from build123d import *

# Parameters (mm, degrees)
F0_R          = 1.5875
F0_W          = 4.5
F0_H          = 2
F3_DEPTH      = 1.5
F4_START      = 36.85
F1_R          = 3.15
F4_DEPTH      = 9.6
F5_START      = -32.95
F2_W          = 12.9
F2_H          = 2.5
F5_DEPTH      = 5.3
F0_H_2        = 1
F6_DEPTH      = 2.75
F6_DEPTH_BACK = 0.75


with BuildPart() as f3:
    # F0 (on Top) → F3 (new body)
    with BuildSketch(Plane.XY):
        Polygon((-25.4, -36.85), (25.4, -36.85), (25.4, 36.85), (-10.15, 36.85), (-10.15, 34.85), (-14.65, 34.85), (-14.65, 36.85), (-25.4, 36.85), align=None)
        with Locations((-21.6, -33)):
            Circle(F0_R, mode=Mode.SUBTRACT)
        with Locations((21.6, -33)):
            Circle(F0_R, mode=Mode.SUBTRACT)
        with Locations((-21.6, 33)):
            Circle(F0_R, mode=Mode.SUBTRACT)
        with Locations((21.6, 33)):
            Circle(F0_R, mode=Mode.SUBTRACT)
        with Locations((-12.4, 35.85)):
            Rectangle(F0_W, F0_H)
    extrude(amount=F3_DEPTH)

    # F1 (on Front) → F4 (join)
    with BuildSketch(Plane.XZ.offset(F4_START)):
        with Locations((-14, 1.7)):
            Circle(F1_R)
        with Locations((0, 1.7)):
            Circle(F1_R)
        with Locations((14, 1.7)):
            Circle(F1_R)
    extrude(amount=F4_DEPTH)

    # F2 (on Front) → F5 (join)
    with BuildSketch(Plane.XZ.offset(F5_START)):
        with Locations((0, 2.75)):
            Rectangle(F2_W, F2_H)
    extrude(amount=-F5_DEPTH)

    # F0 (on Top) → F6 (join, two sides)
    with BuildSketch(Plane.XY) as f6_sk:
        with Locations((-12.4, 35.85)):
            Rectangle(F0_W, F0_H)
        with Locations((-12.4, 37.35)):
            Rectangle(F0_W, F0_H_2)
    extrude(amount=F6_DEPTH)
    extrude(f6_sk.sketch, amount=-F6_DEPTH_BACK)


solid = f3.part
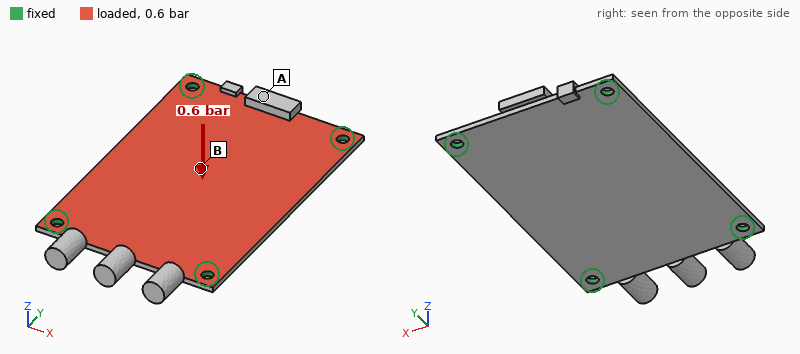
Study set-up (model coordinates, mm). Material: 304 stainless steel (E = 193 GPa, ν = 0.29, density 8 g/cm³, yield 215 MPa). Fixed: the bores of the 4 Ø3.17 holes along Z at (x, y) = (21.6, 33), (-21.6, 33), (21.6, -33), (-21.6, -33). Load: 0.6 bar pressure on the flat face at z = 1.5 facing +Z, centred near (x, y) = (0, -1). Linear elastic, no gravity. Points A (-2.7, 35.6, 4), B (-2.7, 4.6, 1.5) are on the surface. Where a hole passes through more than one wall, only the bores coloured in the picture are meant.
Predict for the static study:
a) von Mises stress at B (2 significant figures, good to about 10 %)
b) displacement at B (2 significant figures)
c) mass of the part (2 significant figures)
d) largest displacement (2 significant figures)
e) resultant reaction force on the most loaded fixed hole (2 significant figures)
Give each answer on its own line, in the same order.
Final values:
28 MPa
76 µm
53 g
79 µm
56 N
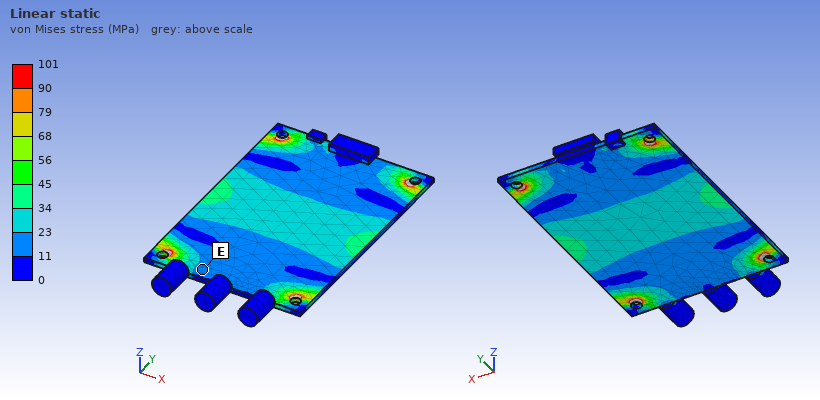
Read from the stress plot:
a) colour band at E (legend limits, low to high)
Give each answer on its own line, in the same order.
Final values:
11 to 23 MPa
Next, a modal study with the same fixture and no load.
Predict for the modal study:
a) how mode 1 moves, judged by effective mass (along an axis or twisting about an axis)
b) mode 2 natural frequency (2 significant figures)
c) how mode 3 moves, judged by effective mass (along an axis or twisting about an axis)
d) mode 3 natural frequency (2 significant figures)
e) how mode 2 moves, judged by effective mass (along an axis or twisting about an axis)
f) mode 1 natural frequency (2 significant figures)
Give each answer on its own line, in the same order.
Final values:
along Z
2300 Hz
twisting about Y
2400 Hz
along Z
1500 Hz
